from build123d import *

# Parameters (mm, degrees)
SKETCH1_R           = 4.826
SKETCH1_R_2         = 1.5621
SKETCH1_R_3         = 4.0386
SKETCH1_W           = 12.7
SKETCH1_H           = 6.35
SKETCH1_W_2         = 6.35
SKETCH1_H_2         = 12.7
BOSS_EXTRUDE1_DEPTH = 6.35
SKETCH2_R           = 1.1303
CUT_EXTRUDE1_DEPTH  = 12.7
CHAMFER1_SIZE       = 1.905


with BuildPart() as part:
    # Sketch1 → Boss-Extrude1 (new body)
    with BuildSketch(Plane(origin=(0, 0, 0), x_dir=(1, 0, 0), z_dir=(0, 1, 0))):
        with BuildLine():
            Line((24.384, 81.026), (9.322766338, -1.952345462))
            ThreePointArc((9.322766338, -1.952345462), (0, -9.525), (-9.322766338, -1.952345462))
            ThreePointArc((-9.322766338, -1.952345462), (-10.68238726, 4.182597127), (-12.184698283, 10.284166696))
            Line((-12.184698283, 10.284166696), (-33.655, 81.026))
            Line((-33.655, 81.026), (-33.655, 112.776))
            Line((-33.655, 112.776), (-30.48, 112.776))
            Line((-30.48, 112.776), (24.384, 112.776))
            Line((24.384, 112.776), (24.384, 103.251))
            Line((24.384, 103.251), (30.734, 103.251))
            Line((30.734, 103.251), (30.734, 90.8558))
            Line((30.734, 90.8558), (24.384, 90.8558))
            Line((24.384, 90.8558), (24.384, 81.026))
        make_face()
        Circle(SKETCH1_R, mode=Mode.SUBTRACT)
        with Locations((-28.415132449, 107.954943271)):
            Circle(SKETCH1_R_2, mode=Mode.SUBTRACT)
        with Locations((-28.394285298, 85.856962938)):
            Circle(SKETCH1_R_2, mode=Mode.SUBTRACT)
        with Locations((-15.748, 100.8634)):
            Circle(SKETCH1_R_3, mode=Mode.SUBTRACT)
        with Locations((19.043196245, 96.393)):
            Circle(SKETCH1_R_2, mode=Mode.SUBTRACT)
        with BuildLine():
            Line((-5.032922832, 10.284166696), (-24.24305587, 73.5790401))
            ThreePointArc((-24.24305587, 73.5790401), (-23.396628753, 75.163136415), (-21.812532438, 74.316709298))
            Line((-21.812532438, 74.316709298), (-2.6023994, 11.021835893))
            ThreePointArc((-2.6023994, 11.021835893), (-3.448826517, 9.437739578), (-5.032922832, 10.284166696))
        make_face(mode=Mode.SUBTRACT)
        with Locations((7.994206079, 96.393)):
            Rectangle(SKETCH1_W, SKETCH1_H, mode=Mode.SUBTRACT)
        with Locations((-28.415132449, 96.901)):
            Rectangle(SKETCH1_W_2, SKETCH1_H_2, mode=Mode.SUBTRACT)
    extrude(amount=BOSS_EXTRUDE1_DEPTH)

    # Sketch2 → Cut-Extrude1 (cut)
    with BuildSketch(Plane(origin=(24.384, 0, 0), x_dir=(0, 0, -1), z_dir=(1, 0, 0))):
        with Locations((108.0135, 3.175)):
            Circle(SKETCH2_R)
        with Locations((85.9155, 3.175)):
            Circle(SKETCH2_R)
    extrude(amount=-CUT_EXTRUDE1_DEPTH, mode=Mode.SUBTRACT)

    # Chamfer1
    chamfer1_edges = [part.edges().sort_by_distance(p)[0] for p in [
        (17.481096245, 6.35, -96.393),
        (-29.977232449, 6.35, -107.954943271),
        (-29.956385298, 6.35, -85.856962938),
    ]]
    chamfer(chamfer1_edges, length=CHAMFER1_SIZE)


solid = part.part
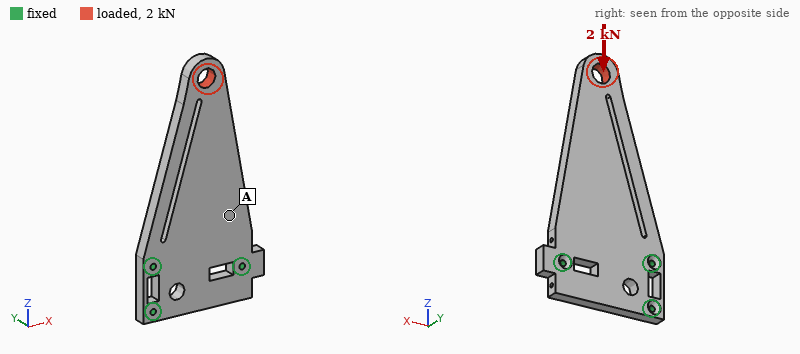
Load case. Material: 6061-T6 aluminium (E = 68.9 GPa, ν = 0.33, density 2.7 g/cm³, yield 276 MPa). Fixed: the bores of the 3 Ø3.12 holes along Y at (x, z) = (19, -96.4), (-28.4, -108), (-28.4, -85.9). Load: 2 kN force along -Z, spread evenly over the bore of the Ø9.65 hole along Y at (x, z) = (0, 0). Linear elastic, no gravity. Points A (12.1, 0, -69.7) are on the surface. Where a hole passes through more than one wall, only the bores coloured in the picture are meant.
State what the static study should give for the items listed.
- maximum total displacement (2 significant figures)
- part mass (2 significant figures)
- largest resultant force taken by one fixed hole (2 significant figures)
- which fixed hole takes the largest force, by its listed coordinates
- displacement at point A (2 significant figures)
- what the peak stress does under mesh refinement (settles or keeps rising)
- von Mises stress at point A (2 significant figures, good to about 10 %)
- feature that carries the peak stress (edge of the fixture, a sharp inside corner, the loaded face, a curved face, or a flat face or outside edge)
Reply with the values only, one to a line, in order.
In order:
27 µm
80 g
1.2 kN
(19, -96.4)
6.2 µm
keeps rising
8.8 MPa
edge of the fixture
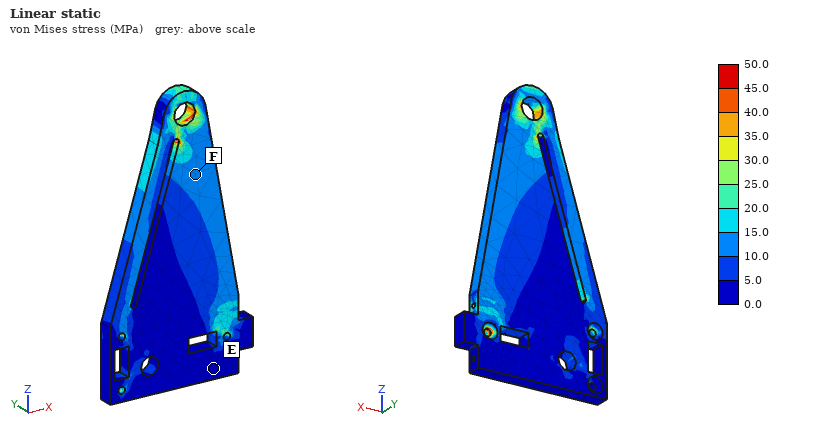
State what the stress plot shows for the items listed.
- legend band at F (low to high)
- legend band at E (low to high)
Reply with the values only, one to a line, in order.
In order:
10.0 to 15.0 MPa
0.0 to 5.0 MPa
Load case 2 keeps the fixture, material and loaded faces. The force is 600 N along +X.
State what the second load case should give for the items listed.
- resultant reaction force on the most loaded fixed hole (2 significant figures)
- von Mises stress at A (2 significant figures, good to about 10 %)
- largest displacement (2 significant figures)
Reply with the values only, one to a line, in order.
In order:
1.1 kN
9.8 MPa
69 µm
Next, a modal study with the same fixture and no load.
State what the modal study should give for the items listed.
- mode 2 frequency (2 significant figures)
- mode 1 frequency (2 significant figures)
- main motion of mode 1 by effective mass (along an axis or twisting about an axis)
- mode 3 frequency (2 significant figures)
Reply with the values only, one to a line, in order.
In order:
3100 Hz
700 Hz
along Y
3700 Hz
